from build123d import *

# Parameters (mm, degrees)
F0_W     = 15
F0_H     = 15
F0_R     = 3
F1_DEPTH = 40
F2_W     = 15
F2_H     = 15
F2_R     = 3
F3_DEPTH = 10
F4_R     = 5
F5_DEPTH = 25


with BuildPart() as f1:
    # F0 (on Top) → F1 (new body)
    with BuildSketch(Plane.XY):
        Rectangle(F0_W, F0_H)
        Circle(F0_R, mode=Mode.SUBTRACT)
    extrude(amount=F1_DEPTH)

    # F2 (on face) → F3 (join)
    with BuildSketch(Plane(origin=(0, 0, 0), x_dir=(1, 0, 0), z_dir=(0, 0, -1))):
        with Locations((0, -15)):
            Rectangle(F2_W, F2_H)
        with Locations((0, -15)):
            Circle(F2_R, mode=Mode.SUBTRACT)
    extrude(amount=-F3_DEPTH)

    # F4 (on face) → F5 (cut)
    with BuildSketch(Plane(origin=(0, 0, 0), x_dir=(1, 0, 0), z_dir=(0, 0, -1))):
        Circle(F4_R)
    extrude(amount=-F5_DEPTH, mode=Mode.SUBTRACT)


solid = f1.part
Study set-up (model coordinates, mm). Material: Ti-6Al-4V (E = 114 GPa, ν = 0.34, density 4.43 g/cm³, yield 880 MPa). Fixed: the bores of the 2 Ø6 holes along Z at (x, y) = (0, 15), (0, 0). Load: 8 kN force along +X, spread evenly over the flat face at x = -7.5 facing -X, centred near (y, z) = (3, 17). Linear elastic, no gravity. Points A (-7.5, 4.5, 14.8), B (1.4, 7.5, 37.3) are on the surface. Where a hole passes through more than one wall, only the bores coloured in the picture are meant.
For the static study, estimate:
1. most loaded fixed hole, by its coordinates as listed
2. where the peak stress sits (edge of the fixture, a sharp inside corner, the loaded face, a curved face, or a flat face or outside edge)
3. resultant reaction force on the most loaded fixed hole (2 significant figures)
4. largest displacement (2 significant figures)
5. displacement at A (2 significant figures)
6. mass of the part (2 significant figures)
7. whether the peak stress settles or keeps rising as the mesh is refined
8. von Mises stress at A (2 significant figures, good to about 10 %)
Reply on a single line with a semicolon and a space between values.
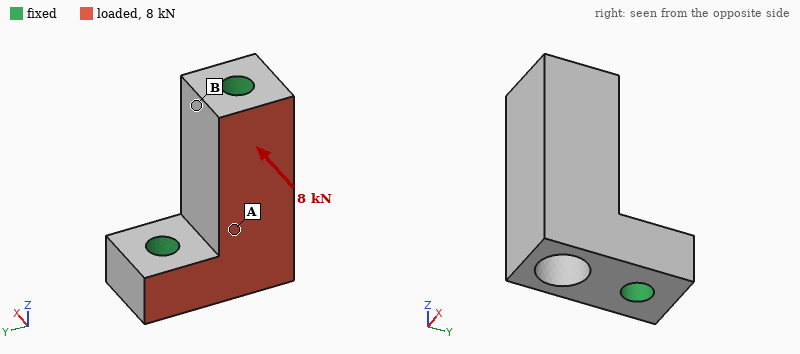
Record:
(0, 0); edge of the fixture; 4.5 kN; 26 µm; 10 µm; 38 g; keeps rising; 30 MPa
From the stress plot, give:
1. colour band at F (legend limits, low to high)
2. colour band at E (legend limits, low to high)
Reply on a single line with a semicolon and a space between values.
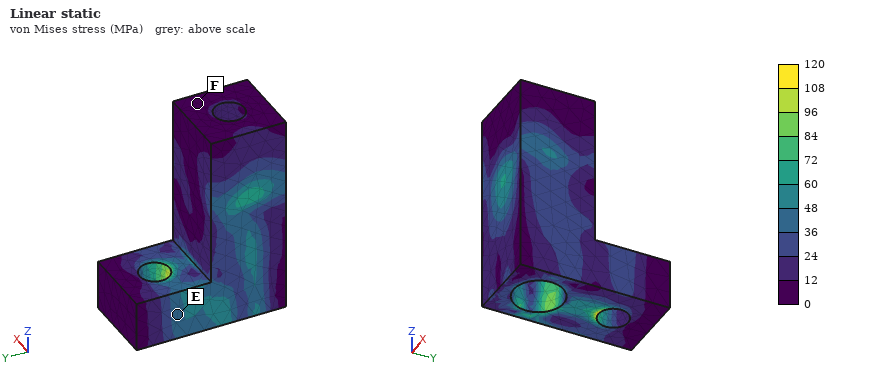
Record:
0 to 12 MPa; 36 to 48 MPa
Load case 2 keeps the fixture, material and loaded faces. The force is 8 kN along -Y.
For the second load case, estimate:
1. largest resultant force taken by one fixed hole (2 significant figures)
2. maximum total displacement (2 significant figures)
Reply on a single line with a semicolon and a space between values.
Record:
4.2 kN; 20 µm
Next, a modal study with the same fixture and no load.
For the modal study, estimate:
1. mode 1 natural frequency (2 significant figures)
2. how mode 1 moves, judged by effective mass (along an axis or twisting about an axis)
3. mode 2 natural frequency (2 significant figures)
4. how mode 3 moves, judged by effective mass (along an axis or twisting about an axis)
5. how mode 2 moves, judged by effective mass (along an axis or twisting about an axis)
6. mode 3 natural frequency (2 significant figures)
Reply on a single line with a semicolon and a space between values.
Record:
20 kHz; along X; 39 kHz; along Z; along Y; 42 kHz
